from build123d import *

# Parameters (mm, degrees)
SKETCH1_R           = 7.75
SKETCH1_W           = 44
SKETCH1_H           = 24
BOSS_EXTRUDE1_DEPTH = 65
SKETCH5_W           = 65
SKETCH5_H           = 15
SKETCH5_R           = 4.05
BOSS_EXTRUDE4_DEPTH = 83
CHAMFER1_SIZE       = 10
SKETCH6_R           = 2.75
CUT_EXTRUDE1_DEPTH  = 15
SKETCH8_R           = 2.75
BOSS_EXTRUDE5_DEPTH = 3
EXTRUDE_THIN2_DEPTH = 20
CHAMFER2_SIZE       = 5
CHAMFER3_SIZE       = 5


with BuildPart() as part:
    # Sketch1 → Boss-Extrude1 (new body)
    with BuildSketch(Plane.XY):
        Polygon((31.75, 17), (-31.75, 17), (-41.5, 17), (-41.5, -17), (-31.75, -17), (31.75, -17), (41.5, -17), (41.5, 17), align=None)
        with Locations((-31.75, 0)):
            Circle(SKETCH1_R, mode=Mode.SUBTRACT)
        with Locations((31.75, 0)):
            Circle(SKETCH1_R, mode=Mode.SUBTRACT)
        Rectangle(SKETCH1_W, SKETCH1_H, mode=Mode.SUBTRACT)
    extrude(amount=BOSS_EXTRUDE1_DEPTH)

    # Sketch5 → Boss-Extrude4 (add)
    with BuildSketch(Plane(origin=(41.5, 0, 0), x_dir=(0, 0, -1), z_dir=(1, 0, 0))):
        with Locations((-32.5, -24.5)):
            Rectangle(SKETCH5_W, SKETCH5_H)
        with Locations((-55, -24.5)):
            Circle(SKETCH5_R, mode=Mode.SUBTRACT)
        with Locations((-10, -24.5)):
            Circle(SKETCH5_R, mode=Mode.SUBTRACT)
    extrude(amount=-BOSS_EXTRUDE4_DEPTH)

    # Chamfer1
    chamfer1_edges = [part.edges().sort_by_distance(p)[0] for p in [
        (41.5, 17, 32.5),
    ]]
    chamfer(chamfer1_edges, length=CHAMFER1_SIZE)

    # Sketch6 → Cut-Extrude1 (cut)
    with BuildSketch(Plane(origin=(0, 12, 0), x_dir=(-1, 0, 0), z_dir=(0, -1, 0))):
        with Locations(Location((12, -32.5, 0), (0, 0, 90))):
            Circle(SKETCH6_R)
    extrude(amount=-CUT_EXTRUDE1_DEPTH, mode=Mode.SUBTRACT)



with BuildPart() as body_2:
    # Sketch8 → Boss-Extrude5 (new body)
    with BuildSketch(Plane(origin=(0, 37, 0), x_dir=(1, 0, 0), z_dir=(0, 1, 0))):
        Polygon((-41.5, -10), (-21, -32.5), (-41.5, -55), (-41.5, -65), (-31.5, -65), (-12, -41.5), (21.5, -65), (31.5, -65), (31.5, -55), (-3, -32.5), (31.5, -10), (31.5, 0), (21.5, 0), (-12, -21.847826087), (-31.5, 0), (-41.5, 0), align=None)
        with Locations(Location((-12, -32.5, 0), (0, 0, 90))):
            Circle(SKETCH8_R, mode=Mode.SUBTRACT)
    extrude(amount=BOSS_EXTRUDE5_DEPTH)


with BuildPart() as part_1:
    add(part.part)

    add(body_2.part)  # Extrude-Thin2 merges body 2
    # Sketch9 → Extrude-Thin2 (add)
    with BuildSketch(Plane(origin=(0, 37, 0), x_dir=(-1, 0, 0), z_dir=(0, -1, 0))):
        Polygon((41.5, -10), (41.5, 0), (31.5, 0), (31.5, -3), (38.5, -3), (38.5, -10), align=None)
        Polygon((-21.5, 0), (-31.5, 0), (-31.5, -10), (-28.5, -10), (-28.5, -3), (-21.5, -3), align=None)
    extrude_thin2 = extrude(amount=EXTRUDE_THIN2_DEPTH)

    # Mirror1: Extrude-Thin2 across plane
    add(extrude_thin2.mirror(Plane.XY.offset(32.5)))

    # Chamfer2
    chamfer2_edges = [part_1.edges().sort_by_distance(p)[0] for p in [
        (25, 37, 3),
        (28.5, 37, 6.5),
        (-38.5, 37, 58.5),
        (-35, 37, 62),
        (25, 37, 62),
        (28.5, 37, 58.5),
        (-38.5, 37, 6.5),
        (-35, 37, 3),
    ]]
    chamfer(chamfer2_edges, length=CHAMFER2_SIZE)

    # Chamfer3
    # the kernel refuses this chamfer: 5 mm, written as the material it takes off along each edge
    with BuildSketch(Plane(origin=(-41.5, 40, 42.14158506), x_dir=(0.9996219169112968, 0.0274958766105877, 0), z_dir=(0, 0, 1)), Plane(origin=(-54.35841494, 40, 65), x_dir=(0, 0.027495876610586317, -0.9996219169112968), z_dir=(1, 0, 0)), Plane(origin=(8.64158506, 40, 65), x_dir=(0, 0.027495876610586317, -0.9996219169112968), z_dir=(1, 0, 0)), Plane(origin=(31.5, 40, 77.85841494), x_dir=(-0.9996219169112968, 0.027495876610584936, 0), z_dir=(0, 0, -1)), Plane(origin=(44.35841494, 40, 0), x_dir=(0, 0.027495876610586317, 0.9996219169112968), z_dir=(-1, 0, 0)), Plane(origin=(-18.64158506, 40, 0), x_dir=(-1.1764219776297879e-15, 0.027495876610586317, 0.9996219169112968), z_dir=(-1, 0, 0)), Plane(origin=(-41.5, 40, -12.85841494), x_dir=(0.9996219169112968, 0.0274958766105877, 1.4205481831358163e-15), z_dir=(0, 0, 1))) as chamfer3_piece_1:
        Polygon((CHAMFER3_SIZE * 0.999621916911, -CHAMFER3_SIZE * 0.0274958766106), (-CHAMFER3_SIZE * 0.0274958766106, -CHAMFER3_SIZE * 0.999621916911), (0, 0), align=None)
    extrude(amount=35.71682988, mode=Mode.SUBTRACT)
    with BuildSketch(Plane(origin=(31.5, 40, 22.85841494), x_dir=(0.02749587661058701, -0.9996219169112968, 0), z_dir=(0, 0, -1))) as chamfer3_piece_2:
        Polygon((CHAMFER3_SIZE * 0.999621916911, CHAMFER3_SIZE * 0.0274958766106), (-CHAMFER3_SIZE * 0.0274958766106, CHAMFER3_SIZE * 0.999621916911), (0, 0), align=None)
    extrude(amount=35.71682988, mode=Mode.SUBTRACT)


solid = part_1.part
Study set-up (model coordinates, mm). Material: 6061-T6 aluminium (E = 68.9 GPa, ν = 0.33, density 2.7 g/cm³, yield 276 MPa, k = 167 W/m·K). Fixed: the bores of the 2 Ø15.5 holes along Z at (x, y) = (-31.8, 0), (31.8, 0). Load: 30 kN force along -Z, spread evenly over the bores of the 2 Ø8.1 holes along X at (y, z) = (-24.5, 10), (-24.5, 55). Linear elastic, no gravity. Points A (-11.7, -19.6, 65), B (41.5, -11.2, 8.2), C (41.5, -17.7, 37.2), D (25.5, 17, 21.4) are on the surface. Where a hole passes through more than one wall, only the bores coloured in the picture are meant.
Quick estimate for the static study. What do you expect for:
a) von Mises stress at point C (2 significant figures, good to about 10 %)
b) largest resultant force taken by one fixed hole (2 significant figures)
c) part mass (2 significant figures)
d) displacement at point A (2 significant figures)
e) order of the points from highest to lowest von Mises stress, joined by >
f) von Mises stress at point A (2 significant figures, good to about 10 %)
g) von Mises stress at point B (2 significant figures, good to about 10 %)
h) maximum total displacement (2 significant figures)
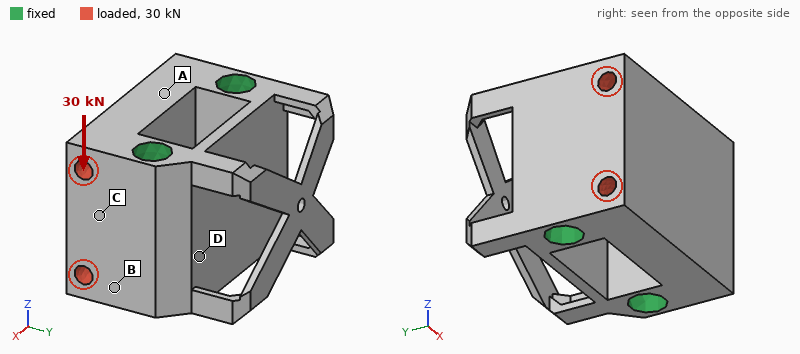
16 MPa
15 kN
460 g
13 µm
C > B > A > D
6.7 MPa
12 MPa
17 µm
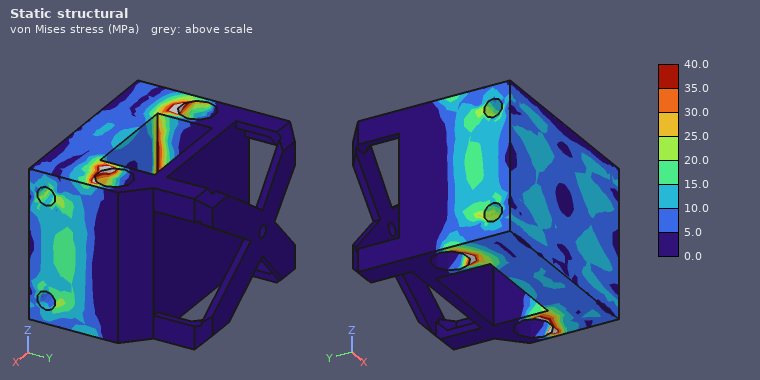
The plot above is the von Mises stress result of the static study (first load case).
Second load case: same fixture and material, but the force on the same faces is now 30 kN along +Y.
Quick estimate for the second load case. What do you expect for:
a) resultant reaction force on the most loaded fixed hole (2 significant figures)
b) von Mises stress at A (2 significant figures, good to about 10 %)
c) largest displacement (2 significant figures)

16 kN
17 MPa
16 µm
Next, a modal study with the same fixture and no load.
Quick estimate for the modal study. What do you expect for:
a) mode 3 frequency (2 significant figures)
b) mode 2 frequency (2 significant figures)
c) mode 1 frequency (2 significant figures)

3900 Hz
3800 Hz
2700 Hz
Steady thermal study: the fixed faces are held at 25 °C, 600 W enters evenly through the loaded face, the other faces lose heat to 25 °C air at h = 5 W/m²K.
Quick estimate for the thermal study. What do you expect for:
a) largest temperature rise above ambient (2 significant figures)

38 K
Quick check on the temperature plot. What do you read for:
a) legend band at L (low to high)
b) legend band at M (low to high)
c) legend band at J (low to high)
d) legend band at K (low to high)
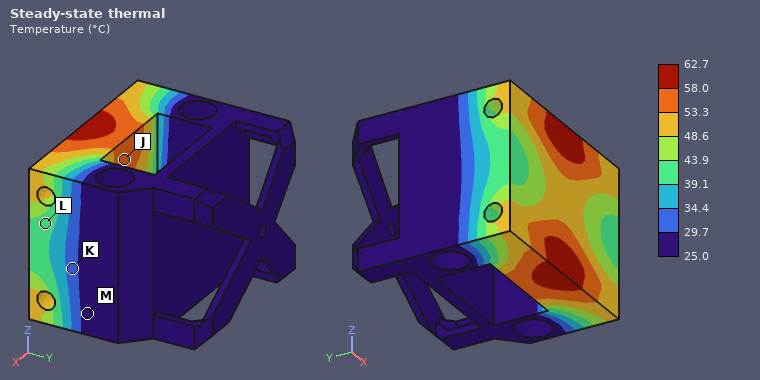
39.1 to 43.9 °C
25.0 to 29.7 °C
53.3 to 58.0 °C
29.7 to 34.4 °C
